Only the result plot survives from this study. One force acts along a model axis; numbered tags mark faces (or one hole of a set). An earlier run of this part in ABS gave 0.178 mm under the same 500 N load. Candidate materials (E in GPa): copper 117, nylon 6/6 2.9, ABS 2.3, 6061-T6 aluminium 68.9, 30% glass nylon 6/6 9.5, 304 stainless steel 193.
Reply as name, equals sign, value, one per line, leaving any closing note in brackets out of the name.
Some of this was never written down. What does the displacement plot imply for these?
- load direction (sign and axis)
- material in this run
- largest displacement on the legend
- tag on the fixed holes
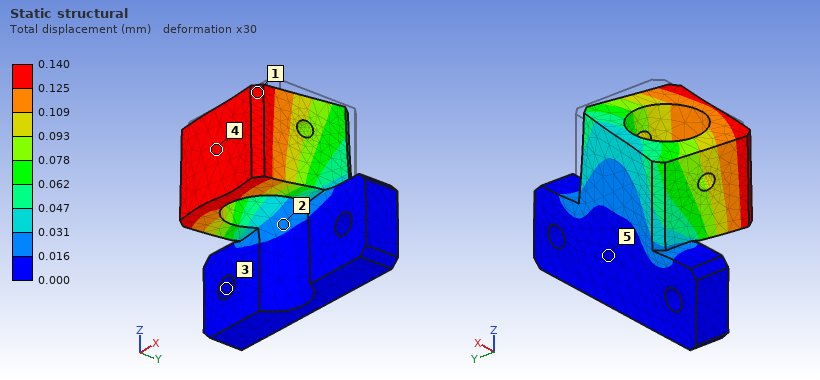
load direction = -X
material in this run = nylon 6/6
largest displacement on the legend = 0.140 mm
tag on the fixed holes = 3
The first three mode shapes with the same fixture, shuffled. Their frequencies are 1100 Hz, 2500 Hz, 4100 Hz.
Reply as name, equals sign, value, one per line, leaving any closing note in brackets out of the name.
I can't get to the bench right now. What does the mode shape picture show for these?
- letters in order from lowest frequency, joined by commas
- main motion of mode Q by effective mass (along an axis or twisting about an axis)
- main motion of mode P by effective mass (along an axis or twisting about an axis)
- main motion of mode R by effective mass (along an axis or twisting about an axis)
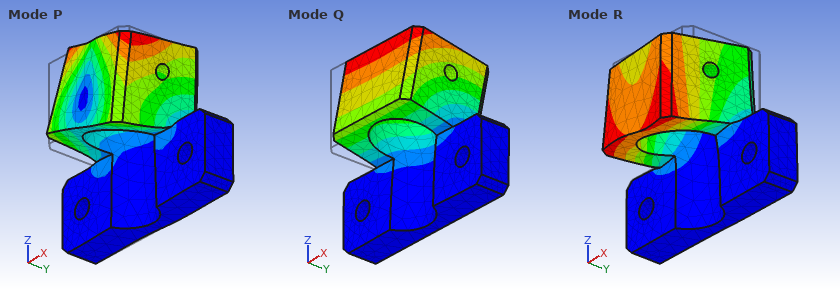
letters in order from lowest frequency, joined by commas = Q, R, P
main motion of mode Q by effective mass = along Y
main motion of mode P by effective mass = along X
main motion of mode R by effective mass = along X
